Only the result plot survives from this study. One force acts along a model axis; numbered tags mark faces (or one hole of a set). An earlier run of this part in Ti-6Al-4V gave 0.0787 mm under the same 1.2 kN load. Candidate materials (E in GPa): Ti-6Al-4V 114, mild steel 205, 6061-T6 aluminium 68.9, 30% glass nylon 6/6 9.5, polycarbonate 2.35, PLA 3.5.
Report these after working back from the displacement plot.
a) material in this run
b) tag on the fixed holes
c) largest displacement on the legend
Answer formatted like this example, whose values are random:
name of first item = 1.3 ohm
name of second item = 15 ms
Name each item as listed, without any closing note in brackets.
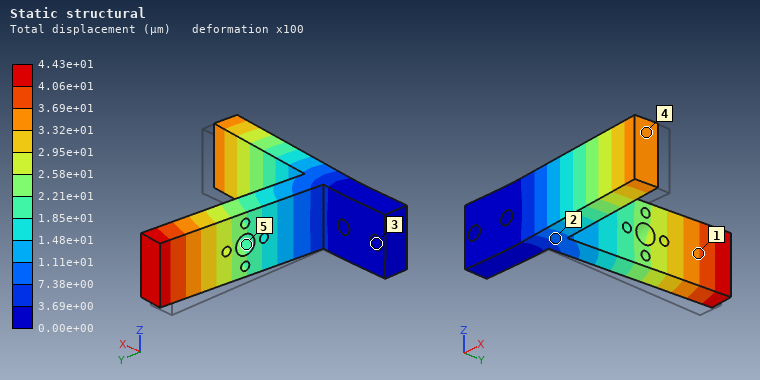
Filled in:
material in this run = mild steel
tag on the fixed holes = 3
largest displacement on the legend = 4.43e+01 µm
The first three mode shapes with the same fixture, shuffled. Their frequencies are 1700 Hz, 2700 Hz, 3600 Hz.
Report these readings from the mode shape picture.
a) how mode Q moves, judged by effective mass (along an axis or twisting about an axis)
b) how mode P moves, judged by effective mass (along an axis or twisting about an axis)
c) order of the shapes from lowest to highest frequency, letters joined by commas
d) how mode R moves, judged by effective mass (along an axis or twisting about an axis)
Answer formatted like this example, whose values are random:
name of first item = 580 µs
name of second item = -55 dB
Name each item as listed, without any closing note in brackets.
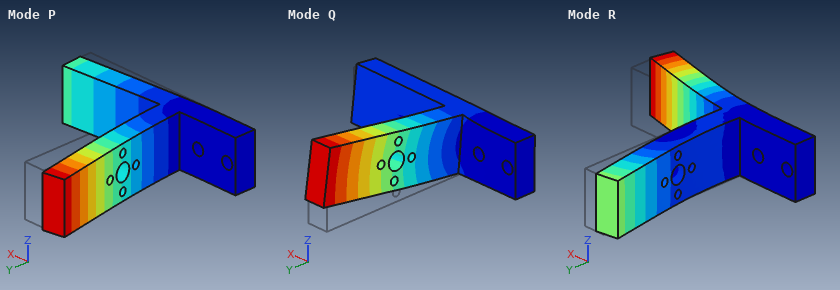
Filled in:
how mode Q moves, judged by effective mass = along Z
how mode P moves, judged by effective mass = along X
order of the shapes from lowest to highest frequency, letters joined by commas = P, Q, R
how mode R moves, judged by effective mass = along Y
